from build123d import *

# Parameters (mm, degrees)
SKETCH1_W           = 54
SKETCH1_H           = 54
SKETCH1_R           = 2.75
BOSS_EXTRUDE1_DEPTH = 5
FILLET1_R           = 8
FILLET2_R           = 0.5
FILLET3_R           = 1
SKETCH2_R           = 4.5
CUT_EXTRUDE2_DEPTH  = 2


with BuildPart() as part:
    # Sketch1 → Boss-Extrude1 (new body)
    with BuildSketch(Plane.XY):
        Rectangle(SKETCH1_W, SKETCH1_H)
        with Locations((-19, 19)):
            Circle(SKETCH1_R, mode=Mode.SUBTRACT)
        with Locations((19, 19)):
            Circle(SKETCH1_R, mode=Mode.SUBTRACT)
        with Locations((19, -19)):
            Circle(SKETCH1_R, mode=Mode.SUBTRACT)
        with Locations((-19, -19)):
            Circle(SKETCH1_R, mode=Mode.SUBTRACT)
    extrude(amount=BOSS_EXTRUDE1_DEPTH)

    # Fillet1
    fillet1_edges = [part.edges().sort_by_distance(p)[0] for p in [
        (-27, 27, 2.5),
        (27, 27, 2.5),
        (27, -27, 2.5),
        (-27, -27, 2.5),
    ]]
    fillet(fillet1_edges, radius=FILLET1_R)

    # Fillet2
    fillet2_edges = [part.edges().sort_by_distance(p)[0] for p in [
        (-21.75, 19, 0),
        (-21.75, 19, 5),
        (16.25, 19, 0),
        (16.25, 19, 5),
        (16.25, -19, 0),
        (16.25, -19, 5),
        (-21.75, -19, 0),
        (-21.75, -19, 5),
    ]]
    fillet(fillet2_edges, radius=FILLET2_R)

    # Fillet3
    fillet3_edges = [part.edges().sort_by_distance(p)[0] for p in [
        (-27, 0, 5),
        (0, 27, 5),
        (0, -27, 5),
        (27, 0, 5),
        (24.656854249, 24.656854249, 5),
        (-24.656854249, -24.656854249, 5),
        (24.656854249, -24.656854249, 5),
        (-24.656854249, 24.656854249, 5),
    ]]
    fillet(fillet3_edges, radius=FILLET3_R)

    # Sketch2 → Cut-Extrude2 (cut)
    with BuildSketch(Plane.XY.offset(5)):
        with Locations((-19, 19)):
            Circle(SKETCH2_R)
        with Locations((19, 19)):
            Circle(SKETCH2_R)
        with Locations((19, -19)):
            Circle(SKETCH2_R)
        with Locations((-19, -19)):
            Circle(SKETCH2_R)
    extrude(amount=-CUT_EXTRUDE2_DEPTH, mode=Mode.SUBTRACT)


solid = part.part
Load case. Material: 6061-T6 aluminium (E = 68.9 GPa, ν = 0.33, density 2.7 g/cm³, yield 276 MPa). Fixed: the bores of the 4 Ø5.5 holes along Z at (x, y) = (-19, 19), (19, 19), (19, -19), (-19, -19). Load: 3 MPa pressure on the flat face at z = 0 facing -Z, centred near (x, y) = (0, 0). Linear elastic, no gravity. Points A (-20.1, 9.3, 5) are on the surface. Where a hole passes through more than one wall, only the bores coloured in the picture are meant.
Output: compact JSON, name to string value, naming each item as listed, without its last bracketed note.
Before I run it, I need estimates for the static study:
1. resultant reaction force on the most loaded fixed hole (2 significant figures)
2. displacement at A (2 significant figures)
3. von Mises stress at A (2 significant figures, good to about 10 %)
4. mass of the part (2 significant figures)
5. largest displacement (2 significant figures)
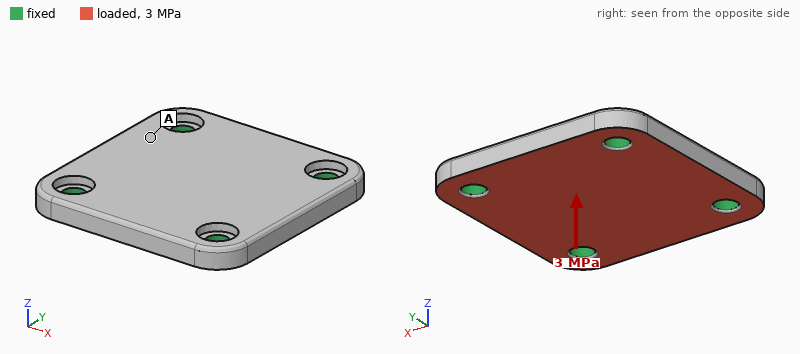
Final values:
{"resultant reaction force on the most loaded fixed hole": "2.2 kN", "displacement at A": "27 µm", "von Mises stress at A": "46 MPa", "mass of the part": "36 g", "largest displacement": "69 µm"}
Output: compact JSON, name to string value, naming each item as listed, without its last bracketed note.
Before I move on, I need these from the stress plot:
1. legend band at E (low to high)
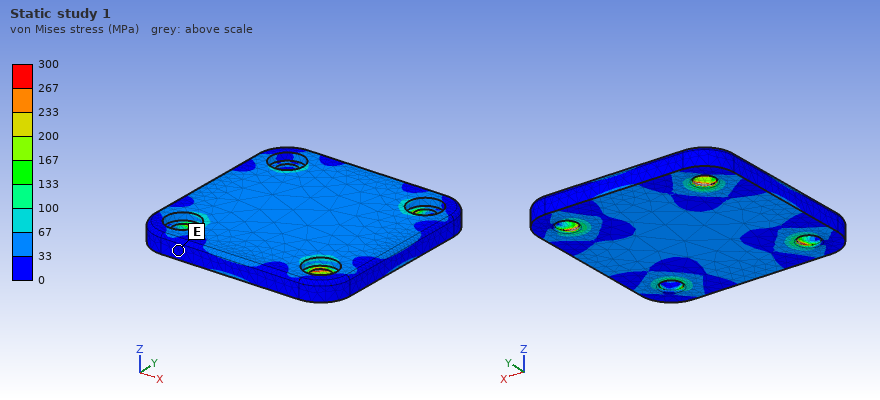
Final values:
{"legend band at E": "0 to 33 MPa"}
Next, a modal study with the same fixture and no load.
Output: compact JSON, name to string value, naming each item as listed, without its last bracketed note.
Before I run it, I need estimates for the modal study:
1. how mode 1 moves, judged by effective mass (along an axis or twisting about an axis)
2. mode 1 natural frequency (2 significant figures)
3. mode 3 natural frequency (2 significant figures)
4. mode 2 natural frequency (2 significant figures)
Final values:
{"how mode 1 moves, judged by effective mass": "along Z", "mode 1 natural frequency": "11 kHz", "mode 3 natural frequency": "15 kHz", "mode 2 natural frequency": "15 kHz"}
